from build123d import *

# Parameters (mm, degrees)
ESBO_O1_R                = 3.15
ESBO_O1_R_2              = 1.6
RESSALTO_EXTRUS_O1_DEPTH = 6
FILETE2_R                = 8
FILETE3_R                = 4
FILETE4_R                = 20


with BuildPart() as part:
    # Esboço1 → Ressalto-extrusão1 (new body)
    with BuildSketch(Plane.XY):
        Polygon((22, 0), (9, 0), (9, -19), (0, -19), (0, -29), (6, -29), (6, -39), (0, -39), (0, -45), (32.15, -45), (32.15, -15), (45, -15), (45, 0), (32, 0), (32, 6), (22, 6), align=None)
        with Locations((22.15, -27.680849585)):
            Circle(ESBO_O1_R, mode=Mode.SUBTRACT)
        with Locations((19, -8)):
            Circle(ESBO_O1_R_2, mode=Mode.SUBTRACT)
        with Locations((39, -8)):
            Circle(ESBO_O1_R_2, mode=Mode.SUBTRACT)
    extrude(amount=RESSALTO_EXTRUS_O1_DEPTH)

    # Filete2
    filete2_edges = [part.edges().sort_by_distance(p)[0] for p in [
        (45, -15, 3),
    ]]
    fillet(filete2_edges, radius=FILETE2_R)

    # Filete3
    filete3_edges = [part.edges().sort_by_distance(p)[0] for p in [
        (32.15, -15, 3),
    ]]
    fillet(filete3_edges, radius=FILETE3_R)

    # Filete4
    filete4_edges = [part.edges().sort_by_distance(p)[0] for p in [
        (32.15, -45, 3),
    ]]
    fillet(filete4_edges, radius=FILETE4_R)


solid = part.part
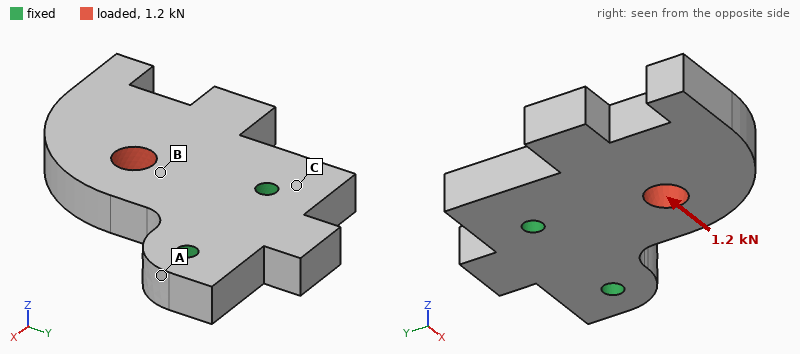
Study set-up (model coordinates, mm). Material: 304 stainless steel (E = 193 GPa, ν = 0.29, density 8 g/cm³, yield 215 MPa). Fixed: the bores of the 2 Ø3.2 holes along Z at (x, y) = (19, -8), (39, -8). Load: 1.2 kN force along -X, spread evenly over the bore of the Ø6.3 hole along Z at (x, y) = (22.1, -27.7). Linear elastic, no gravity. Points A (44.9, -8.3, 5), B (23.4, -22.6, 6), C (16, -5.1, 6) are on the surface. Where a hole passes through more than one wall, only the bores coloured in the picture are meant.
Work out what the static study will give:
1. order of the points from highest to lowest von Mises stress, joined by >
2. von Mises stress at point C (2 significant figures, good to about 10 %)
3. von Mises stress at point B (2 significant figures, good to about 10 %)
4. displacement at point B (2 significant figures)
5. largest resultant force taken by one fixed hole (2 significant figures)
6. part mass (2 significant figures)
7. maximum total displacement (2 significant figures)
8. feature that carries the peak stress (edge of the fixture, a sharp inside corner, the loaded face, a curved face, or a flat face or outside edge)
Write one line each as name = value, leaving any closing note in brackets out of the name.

order of the points from highest to lowest von Mises stress, joined by > = B > C > A
von Mises stress at point C = 18 MPa
von Mises stress at point B = 32 MPa
displacement at point B = 4.0 µm
largest resultant force taken by one fixed hole = 1.2 kN
part mass = 64 g
maximum total displacement = 13 µm
feature that carries the peak stress = edge of the fixture
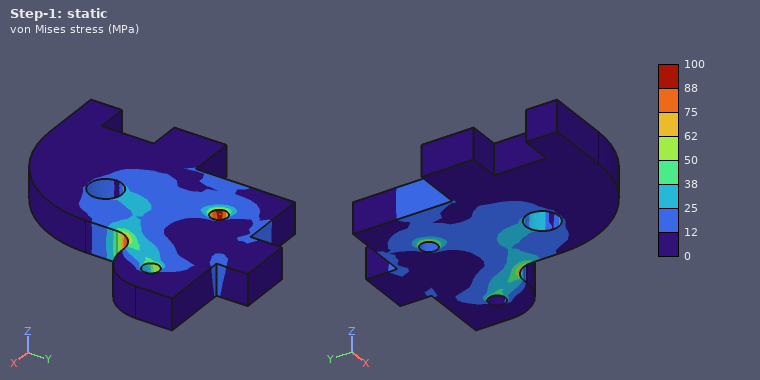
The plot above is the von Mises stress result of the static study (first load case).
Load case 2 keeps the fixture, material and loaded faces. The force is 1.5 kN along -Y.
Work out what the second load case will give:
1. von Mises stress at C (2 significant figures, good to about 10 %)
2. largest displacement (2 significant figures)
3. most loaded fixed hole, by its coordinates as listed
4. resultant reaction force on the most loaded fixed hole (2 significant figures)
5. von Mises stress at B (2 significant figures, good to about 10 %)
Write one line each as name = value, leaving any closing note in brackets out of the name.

von Mises stress at C = 7.5 MPa
largest displacement = 2.0 µm
most loaded fixed hole, by its coordinates as listed = (19, -8)
resultant reaction force on the most loaded fixed hole = 1.2 kN
von Mises stress at B = 15 MPa
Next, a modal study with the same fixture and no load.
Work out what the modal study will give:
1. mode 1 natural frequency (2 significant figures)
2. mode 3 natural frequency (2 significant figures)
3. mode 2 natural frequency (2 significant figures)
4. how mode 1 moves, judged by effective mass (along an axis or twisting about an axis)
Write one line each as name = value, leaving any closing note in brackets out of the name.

mode 1 natural frequency = 3200 Hz
mode 3 natural frequency = 8800 Hz
mode 2 natural frequency = 8700 Hz
how mode 1 moves, judged by effective mass = along Z
